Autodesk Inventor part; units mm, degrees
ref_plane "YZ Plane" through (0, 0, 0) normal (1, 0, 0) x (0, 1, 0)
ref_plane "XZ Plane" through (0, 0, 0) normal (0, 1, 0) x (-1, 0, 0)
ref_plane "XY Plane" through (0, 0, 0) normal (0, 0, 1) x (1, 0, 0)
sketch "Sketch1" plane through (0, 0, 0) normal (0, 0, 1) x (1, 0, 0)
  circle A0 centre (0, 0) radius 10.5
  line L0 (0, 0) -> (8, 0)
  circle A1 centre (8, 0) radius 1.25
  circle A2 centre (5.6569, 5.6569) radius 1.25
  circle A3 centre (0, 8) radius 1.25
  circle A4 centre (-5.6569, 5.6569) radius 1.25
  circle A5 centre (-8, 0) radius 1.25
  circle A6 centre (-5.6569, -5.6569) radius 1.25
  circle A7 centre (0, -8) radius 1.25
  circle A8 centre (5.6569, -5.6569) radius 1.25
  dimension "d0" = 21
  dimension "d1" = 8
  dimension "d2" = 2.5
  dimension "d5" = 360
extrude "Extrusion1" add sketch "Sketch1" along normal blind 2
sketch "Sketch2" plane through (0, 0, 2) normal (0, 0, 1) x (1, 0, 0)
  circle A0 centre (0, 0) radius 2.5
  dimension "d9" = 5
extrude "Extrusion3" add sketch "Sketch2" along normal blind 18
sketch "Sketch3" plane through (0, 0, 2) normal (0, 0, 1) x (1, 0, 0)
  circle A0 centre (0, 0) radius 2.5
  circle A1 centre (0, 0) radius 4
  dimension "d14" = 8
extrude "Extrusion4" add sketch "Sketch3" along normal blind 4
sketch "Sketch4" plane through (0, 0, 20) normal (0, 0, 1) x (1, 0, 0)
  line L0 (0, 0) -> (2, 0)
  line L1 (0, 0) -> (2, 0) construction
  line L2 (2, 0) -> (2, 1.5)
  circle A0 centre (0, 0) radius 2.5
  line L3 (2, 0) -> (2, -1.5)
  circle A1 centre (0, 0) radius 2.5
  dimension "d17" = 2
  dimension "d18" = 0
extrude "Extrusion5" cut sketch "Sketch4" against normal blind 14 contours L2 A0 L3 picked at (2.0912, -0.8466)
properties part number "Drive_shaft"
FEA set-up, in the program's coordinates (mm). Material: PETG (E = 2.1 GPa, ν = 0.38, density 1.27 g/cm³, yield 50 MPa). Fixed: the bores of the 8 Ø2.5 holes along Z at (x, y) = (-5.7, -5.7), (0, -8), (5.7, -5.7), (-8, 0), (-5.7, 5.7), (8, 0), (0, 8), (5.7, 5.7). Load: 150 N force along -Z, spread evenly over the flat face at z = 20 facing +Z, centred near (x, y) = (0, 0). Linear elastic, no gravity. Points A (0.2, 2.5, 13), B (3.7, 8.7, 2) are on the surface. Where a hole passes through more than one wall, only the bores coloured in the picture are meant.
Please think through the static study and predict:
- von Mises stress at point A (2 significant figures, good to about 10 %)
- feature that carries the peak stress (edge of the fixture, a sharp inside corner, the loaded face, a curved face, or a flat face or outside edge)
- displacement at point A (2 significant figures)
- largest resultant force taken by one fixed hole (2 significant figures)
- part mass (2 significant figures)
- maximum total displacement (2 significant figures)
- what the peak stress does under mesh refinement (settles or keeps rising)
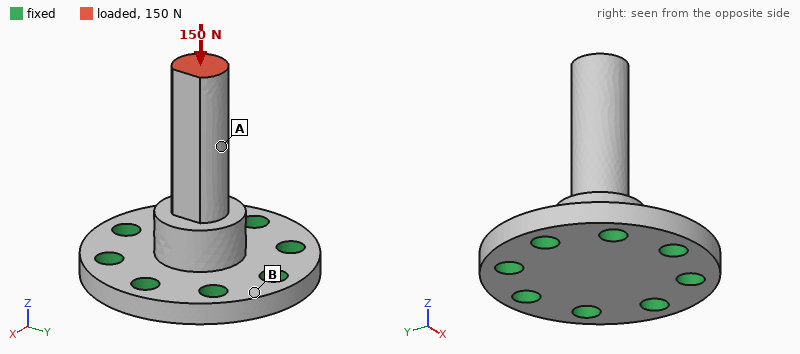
8.1 MPa
edge of the fixture
64 µm
22 N
1.4 g
92 µm
keeps rising
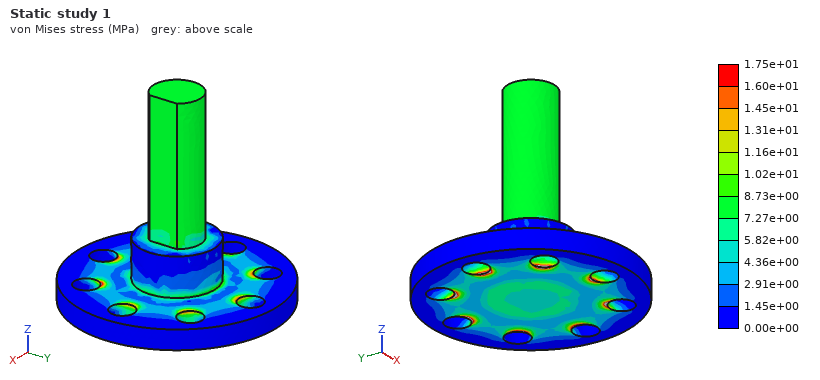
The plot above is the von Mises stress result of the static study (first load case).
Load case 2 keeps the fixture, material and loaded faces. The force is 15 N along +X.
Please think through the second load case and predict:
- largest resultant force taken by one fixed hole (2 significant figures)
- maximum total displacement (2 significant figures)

13 N
0.42 mm
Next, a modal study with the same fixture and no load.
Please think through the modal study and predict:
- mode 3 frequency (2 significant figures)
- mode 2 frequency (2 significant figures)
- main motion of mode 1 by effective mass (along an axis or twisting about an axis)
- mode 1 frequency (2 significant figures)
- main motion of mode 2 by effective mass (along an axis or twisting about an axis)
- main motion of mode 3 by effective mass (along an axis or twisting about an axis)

12 kHz
3200 Hz
along X
3000 Hz
along Y
along Z
